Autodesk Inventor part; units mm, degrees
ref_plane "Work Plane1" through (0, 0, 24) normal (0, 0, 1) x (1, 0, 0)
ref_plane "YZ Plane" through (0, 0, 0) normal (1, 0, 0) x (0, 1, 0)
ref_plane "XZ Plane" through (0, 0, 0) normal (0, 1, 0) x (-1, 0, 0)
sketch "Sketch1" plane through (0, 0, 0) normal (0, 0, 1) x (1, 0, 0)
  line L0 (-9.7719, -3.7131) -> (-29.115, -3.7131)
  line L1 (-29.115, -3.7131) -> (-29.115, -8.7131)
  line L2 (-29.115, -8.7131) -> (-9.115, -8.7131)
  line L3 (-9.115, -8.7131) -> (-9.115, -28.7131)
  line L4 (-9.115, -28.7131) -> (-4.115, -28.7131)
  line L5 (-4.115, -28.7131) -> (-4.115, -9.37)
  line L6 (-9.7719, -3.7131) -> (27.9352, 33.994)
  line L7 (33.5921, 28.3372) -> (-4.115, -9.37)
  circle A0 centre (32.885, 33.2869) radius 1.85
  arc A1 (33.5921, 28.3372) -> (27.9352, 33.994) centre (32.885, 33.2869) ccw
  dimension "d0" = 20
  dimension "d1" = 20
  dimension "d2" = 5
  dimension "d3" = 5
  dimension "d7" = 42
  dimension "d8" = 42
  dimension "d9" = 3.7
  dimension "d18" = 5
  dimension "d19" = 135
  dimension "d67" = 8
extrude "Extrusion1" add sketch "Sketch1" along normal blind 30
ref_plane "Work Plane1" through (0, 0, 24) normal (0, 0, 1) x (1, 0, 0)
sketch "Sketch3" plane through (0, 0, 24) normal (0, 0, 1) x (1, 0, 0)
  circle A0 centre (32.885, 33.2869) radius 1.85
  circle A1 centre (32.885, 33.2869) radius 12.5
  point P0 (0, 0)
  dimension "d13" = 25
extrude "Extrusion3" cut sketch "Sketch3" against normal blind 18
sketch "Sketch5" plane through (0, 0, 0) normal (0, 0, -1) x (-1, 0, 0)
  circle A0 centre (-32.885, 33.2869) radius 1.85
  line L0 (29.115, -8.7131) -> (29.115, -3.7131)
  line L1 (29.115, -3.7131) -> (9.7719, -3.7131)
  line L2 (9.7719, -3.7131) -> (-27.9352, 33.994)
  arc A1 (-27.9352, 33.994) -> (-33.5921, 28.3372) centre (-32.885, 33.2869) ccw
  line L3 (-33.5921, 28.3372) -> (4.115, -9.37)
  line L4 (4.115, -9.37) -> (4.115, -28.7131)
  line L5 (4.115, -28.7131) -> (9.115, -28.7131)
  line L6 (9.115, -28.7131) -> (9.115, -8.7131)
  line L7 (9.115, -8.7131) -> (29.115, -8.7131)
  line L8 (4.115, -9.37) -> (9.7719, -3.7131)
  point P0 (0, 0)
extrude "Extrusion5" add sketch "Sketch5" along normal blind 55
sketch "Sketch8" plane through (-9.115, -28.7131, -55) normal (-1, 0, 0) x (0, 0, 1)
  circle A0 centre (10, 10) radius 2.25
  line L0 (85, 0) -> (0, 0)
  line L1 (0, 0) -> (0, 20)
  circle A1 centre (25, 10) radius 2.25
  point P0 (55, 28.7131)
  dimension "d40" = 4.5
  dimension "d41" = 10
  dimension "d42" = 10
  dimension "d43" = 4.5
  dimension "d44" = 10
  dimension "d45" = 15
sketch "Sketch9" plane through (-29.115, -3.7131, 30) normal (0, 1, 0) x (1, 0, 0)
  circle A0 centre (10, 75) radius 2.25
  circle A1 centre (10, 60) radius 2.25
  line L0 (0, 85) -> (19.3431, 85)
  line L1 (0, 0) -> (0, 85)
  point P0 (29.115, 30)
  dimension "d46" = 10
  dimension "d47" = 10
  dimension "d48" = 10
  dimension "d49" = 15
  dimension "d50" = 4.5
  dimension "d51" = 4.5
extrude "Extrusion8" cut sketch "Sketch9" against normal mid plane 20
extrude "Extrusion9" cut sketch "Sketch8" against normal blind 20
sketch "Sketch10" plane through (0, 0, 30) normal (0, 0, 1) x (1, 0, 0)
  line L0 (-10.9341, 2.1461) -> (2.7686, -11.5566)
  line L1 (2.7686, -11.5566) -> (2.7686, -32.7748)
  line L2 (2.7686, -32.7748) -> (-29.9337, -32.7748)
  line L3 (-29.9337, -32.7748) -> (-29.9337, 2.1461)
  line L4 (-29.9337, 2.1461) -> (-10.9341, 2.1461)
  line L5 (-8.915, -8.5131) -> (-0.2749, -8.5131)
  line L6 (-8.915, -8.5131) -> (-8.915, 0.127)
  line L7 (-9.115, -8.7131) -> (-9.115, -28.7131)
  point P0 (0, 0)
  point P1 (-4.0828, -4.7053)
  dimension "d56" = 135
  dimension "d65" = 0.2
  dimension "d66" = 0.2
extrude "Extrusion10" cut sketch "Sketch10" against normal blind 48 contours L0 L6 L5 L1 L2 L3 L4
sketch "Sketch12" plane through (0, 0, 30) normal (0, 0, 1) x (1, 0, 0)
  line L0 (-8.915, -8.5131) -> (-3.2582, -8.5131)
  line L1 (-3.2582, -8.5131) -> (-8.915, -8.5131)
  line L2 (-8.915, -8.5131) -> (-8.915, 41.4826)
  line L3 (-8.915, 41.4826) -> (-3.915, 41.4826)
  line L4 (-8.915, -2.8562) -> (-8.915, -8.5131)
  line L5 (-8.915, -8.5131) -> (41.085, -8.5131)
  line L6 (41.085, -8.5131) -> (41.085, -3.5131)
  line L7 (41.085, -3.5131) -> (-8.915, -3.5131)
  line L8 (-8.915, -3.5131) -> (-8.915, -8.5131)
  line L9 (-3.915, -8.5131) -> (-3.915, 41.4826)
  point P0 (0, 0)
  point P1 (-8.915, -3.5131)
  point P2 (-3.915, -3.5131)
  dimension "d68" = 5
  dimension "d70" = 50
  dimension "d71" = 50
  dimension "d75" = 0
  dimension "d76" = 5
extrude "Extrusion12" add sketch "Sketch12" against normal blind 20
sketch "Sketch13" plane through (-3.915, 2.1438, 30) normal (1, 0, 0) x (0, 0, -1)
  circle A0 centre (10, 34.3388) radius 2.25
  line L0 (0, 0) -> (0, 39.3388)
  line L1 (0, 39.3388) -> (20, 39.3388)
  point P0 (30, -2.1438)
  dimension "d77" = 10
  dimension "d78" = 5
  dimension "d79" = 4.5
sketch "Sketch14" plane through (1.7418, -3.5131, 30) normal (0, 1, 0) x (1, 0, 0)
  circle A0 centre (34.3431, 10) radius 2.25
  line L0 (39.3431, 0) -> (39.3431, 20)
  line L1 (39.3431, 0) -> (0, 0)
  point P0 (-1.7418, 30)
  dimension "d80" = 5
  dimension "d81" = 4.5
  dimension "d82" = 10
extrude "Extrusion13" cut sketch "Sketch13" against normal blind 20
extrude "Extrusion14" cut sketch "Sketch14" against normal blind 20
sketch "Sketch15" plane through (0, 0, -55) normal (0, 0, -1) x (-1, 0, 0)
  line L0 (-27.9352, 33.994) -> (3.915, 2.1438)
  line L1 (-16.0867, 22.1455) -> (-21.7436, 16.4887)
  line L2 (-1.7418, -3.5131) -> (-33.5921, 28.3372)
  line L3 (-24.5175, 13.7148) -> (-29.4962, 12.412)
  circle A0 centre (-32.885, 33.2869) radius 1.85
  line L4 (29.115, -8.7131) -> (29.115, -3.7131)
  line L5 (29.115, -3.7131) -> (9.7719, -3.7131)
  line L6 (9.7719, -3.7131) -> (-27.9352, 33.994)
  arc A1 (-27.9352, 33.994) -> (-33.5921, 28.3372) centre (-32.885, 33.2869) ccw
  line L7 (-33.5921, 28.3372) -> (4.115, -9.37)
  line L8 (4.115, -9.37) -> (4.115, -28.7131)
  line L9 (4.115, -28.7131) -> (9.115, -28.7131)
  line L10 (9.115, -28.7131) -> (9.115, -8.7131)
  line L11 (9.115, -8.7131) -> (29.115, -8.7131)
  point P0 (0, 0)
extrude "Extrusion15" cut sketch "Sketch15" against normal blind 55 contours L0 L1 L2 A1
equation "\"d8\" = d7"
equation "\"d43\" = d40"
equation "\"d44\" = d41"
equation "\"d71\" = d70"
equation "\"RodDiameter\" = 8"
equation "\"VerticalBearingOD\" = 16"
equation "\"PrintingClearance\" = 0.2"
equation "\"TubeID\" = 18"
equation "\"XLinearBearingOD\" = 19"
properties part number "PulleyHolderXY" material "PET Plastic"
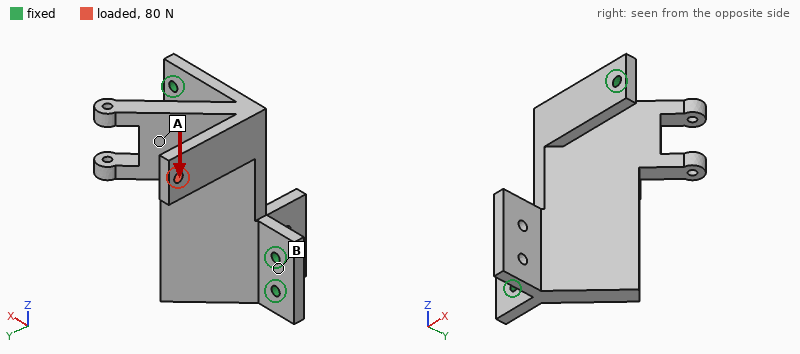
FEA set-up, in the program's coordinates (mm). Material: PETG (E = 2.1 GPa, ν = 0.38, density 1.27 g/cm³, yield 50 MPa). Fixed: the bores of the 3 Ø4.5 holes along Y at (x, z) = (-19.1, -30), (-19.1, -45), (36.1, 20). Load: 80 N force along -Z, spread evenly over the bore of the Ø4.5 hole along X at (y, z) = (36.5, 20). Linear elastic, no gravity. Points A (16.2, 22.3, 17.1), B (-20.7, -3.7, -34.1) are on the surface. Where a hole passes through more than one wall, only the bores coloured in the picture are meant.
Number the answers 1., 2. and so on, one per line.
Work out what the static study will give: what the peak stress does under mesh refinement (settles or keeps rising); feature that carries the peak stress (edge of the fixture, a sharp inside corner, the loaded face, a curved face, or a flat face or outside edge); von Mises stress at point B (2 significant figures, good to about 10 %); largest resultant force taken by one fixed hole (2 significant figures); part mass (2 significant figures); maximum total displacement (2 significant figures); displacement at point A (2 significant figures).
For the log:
1. keeps rising
2. edge of the fixture
3. 1.9 MPa
4. 240 N
5. 56 g
6. 1.3 mm
7. 0.43 mm
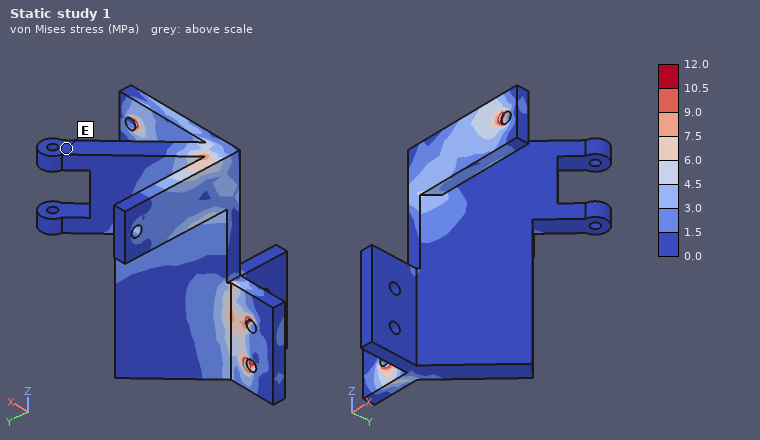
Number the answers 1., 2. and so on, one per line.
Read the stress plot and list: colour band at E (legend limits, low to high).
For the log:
1. 0.0 to 1.5 MPa
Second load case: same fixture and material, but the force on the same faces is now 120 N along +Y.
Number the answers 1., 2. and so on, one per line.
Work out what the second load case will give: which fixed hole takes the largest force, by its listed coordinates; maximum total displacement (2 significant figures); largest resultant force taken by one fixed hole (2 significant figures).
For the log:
1. (-19.1, -30)
2. 1.5 mm
3. 320 N
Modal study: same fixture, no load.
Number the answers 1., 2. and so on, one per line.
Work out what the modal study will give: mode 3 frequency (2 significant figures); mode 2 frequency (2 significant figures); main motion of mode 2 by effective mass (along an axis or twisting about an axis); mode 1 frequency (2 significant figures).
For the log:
1. 600 Hz
2. 400 Hz
3. along Y
4. 320 Hz
